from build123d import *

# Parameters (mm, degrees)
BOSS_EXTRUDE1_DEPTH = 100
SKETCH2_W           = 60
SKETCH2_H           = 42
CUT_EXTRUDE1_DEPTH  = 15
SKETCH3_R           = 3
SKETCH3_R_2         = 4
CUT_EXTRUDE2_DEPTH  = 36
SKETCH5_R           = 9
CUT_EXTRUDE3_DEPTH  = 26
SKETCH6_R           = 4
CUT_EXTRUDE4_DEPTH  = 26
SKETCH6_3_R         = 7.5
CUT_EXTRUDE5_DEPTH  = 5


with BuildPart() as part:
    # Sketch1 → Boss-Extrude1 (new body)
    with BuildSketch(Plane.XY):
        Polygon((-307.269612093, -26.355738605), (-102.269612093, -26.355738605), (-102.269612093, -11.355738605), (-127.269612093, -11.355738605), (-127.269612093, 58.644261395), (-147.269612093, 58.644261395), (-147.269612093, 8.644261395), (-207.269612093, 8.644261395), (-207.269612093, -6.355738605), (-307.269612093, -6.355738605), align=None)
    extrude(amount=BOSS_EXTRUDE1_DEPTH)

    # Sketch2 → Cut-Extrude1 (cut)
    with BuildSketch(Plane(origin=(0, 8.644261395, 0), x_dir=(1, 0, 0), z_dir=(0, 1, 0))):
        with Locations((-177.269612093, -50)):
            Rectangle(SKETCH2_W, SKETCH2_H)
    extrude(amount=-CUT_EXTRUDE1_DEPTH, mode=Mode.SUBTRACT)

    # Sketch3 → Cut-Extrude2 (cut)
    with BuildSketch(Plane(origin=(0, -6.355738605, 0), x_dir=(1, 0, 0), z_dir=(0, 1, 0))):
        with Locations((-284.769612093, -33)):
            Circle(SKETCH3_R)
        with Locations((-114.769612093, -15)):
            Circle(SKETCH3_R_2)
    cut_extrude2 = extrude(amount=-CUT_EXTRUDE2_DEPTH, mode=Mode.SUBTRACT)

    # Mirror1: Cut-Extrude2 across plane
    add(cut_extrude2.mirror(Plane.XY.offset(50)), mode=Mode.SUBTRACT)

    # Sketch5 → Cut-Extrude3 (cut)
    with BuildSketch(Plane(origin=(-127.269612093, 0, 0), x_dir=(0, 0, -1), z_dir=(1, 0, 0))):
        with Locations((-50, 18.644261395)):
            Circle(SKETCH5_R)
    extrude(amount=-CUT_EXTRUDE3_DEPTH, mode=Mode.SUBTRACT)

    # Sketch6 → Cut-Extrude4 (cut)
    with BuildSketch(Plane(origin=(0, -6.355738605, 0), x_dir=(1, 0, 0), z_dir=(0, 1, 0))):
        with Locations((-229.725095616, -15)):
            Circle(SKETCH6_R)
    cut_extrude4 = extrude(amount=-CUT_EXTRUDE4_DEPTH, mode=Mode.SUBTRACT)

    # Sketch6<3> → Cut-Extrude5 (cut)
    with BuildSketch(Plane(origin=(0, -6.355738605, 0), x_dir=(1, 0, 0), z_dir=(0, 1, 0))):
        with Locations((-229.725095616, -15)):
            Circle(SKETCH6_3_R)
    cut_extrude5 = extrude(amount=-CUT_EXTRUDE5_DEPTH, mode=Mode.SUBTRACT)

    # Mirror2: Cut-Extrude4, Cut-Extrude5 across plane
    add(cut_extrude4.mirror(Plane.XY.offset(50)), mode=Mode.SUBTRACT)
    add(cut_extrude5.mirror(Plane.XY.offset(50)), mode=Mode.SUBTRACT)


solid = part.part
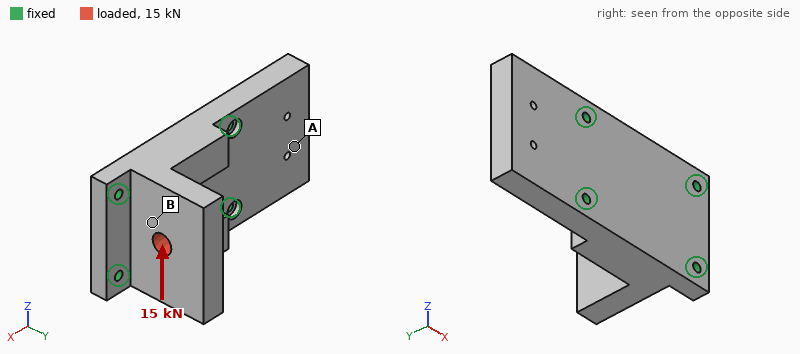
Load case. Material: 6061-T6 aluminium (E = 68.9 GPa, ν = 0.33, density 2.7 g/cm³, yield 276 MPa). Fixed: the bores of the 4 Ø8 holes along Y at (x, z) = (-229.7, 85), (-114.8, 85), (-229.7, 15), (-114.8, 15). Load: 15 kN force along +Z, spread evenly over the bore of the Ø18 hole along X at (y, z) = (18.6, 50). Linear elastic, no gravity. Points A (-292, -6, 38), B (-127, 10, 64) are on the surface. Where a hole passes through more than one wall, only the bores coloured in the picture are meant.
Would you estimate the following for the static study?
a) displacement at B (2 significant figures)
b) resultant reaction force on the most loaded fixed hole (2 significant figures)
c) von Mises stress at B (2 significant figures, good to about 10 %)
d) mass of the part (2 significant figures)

27 µm
8.4 kN
15 MPa
1.5 kg
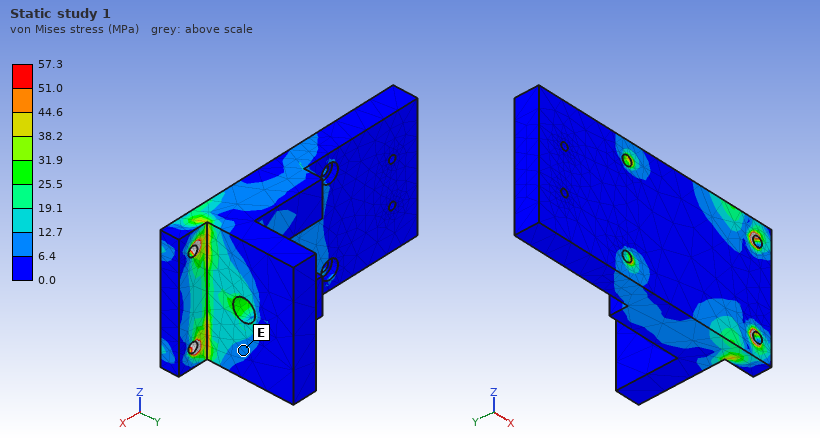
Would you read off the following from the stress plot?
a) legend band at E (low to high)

6.4 to 12.7 MPa
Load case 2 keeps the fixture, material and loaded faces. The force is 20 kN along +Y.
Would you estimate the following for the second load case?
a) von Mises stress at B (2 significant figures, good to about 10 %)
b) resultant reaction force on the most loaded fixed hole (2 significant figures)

16 MPa
8.7 kN
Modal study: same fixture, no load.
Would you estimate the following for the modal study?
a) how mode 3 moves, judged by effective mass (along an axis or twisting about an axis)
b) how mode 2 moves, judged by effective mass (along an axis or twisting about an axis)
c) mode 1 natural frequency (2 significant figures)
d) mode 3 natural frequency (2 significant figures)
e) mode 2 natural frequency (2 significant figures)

along Z
along X
2100 Hz
4000 Hz
3300 Hz
